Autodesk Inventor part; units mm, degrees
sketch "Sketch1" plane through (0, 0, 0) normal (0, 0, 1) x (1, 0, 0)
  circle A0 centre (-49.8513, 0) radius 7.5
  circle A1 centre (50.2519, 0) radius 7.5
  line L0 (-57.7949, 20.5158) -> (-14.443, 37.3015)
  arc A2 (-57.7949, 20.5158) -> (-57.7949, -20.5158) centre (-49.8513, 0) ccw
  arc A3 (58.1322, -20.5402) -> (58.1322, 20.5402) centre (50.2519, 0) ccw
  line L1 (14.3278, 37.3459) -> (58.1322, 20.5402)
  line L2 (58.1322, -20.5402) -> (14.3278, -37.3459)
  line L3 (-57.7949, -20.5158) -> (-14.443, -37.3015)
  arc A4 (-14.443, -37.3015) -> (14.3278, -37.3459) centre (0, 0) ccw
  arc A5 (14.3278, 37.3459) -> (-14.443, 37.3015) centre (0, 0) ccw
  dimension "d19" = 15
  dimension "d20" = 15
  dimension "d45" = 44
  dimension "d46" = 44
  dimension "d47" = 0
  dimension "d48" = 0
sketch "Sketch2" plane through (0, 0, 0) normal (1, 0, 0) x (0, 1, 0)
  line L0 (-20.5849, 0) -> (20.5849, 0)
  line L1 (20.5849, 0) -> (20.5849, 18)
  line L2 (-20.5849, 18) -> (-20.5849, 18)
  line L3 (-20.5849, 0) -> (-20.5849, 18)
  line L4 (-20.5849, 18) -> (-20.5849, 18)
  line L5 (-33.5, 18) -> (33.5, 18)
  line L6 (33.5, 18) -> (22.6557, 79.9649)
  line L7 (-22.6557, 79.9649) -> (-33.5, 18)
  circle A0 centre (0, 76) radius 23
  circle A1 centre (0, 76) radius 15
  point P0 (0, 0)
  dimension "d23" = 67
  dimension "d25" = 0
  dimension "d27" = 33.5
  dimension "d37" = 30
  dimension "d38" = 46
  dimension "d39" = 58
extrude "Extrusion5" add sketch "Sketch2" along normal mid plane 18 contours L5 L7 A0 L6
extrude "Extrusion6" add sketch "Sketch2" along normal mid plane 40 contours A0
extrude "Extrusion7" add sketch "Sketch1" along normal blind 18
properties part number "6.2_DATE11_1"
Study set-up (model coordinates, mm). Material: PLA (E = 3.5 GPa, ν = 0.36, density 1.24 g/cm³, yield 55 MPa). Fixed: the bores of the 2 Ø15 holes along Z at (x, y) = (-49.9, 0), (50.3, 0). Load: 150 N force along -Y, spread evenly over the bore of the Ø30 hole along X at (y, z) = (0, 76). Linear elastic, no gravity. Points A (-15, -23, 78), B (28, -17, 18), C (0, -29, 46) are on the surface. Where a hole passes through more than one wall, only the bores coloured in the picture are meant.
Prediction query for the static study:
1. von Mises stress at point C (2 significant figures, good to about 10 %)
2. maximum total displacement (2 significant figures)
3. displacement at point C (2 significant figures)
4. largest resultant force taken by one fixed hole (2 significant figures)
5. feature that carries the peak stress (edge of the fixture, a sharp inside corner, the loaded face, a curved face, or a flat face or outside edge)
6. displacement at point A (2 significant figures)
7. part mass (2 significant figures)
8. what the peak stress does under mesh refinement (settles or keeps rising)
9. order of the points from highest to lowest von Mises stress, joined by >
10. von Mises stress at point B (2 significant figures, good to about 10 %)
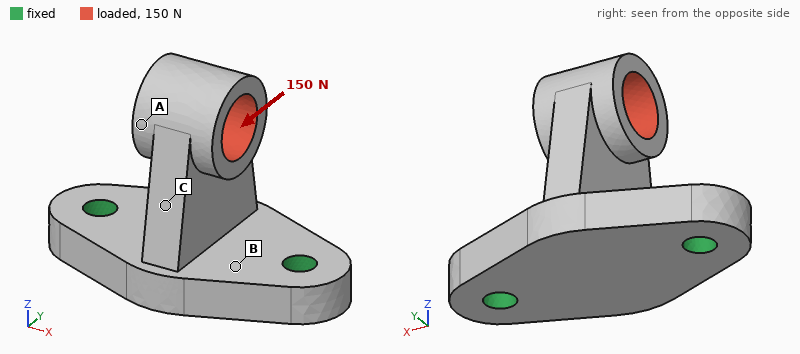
0.57 MPa
0.15 mm
0.068 mm
75 N
edge of the fixture
0.12 mm
280 g
keeps rising
B > C > A
1.0 MPa
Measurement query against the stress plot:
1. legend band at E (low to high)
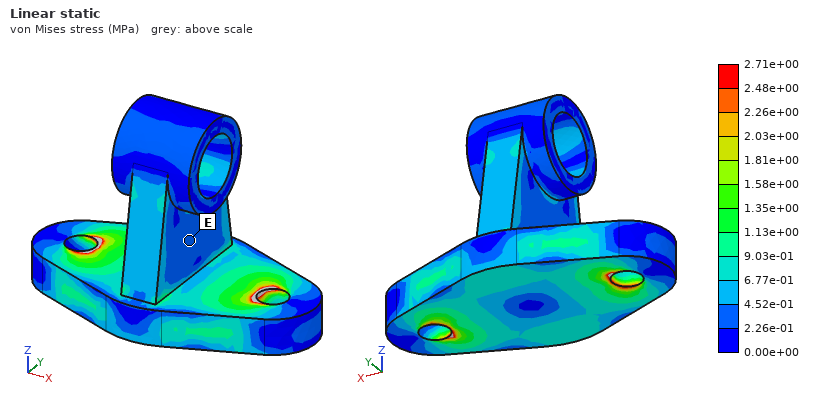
2.26e-01 to 4.52e-01 MPa
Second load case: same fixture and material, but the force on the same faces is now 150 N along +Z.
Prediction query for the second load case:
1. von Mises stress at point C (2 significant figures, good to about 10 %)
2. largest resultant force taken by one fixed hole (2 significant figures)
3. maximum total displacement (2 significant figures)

0.17 MPa
76 N
13 µm
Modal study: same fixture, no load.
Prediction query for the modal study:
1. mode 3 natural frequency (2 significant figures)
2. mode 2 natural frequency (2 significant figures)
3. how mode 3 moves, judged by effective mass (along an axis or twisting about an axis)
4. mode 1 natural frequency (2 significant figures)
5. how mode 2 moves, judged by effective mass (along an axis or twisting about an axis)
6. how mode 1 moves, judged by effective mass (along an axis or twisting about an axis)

1600 Hz
700 Hz
along Z
650 Hz
along Y
along X
